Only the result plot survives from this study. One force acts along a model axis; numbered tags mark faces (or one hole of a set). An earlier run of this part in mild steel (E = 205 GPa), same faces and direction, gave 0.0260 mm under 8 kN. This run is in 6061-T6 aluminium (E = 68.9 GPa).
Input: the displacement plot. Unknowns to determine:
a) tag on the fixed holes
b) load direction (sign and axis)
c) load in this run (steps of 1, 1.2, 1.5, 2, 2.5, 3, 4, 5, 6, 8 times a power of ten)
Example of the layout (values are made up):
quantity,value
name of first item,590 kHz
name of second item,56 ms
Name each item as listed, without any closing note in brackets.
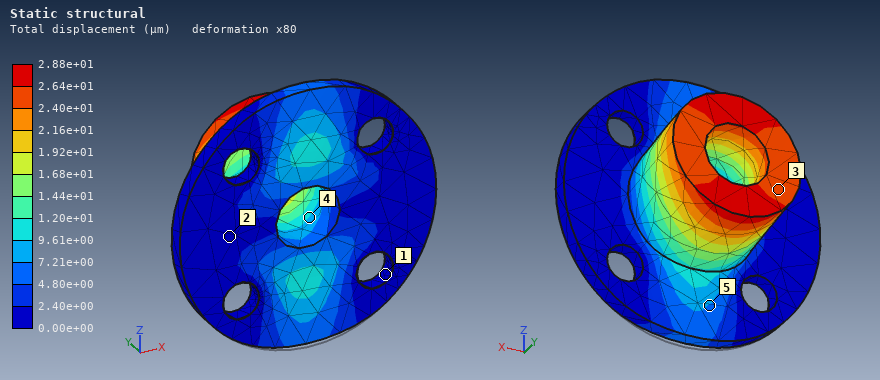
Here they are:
quantity,value
tag on the fixed holes,1
load direction,+Z
load in this run,3 kN
